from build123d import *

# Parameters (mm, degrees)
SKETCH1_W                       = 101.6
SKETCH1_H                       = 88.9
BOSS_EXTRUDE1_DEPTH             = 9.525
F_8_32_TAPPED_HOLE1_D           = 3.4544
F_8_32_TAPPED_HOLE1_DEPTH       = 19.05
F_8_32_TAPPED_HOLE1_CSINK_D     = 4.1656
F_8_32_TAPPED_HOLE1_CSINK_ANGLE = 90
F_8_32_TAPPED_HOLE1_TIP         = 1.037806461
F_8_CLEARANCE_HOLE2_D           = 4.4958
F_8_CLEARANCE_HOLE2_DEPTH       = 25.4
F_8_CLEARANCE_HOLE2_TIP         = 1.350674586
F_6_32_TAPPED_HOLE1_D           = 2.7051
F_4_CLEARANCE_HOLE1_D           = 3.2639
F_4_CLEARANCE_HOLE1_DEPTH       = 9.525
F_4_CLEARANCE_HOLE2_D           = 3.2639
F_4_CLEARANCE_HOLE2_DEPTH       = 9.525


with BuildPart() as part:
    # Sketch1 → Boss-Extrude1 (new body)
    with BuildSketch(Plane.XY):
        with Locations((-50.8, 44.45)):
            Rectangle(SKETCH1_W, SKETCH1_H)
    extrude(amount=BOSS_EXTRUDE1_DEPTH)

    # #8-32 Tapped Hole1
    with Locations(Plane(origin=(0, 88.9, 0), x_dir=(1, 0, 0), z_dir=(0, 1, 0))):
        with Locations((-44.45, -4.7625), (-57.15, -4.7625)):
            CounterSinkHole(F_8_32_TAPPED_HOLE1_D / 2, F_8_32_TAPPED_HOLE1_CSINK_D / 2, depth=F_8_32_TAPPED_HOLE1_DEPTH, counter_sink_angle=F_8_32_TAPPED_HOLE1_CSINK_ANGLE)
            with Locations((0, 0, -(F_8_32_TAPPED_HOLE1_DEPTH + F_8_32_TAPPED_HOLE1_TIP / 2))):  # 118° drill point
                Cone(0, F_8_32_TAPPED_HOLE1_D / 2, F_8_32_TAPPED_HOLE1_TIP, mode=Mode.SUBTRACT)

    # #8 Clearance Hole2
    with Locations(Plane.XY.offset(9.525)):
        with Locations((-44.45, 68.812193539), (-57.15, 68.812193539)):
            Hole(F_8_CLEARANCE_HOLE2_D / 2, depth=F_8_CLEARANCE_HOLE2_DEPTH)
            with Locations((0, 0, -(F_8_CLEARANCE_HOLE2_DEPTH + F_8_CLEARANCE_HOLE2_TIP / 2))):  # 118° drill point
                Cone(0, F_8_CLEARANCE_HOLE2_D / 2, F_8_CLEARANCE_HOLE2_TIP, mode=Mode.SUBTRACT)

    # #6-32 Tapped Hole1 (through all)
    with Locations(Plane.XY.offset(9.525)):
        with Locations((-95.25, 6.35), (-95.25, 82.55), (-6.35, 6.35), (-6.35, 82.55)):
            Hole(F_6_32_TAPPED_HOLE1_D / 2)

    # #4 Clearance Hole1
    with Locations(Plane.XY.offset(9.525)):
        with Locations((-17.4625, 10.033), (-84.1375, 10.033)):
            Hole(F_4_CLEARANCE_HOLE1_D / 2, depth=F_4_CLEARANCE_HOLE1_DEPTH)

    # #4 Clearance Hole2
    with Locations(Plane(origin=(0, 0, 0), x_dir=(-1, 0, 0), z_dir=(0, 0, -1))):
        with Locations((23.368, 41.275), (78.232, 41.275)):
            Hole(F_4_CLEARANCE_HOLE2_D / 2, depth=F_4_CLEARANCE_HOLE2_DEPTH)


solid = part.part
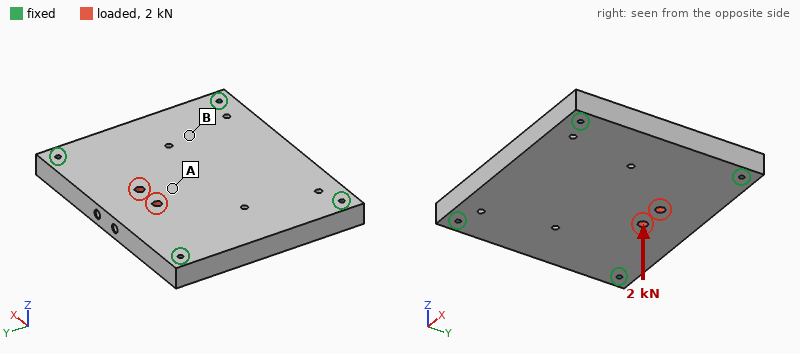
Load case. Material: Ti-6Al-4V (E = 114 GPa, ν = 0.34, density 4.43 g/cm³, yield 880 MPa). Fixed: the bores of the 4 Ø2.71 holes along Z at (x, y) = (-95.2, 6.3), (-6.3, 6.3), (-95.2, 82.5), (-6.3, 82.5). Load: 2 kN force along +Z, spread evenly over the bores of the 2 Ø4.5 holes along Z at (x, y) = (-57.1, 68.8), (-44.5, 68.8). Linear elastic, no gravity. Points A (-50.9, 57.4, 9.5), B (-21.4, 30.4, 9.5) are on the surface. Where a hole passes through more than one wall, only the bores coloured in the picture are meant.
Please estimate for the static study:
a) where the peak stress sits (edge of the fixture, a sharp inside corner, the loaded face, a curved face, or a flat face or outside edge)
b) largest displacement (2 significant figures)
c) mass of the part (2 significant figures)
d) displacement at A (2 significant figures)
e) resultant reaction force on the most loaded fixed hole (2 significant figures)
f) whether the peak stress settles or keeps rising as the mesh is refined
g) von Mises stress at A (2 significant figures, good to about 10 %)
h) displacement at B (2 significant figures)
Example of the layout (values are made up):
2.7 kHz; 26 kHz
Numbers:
edge of the fixture; 32 µm; 380 g; 27 µm; 830 N; keeps rising; 22 MPa; 9.1 µm
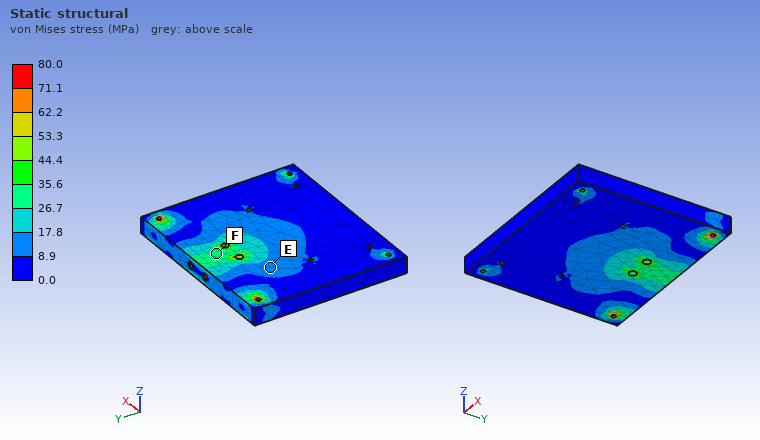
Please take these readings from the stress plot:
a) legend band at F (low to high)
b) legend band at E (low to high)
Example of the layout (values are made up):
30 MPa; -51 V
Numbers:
26.7 to 35.6 MPa; 8.9 to 17.8 MPa
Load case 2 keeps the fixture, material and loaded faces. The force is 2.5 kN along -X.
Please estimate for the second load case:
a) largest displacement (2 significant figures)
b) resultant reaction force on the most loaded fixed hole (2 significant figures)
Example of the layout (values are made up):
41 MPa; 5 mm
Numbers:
2.7 µm; 920 N
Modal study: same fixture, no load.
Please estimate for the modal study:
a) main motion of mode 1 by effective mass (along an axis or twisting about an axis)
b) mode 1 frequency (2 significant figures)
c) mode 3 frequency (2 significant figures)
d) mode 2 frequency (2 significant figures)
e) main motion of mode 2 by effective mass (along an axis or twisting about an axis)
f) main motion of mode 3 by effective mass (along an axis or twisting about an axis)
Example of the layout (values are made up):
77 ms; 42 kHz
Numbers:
along Z; 3800 Hz; 7200 Hz; 6200 Hz; twisting about X; twisting about Y
